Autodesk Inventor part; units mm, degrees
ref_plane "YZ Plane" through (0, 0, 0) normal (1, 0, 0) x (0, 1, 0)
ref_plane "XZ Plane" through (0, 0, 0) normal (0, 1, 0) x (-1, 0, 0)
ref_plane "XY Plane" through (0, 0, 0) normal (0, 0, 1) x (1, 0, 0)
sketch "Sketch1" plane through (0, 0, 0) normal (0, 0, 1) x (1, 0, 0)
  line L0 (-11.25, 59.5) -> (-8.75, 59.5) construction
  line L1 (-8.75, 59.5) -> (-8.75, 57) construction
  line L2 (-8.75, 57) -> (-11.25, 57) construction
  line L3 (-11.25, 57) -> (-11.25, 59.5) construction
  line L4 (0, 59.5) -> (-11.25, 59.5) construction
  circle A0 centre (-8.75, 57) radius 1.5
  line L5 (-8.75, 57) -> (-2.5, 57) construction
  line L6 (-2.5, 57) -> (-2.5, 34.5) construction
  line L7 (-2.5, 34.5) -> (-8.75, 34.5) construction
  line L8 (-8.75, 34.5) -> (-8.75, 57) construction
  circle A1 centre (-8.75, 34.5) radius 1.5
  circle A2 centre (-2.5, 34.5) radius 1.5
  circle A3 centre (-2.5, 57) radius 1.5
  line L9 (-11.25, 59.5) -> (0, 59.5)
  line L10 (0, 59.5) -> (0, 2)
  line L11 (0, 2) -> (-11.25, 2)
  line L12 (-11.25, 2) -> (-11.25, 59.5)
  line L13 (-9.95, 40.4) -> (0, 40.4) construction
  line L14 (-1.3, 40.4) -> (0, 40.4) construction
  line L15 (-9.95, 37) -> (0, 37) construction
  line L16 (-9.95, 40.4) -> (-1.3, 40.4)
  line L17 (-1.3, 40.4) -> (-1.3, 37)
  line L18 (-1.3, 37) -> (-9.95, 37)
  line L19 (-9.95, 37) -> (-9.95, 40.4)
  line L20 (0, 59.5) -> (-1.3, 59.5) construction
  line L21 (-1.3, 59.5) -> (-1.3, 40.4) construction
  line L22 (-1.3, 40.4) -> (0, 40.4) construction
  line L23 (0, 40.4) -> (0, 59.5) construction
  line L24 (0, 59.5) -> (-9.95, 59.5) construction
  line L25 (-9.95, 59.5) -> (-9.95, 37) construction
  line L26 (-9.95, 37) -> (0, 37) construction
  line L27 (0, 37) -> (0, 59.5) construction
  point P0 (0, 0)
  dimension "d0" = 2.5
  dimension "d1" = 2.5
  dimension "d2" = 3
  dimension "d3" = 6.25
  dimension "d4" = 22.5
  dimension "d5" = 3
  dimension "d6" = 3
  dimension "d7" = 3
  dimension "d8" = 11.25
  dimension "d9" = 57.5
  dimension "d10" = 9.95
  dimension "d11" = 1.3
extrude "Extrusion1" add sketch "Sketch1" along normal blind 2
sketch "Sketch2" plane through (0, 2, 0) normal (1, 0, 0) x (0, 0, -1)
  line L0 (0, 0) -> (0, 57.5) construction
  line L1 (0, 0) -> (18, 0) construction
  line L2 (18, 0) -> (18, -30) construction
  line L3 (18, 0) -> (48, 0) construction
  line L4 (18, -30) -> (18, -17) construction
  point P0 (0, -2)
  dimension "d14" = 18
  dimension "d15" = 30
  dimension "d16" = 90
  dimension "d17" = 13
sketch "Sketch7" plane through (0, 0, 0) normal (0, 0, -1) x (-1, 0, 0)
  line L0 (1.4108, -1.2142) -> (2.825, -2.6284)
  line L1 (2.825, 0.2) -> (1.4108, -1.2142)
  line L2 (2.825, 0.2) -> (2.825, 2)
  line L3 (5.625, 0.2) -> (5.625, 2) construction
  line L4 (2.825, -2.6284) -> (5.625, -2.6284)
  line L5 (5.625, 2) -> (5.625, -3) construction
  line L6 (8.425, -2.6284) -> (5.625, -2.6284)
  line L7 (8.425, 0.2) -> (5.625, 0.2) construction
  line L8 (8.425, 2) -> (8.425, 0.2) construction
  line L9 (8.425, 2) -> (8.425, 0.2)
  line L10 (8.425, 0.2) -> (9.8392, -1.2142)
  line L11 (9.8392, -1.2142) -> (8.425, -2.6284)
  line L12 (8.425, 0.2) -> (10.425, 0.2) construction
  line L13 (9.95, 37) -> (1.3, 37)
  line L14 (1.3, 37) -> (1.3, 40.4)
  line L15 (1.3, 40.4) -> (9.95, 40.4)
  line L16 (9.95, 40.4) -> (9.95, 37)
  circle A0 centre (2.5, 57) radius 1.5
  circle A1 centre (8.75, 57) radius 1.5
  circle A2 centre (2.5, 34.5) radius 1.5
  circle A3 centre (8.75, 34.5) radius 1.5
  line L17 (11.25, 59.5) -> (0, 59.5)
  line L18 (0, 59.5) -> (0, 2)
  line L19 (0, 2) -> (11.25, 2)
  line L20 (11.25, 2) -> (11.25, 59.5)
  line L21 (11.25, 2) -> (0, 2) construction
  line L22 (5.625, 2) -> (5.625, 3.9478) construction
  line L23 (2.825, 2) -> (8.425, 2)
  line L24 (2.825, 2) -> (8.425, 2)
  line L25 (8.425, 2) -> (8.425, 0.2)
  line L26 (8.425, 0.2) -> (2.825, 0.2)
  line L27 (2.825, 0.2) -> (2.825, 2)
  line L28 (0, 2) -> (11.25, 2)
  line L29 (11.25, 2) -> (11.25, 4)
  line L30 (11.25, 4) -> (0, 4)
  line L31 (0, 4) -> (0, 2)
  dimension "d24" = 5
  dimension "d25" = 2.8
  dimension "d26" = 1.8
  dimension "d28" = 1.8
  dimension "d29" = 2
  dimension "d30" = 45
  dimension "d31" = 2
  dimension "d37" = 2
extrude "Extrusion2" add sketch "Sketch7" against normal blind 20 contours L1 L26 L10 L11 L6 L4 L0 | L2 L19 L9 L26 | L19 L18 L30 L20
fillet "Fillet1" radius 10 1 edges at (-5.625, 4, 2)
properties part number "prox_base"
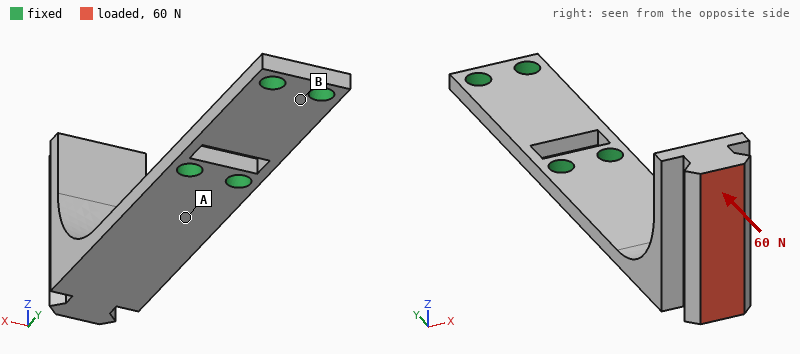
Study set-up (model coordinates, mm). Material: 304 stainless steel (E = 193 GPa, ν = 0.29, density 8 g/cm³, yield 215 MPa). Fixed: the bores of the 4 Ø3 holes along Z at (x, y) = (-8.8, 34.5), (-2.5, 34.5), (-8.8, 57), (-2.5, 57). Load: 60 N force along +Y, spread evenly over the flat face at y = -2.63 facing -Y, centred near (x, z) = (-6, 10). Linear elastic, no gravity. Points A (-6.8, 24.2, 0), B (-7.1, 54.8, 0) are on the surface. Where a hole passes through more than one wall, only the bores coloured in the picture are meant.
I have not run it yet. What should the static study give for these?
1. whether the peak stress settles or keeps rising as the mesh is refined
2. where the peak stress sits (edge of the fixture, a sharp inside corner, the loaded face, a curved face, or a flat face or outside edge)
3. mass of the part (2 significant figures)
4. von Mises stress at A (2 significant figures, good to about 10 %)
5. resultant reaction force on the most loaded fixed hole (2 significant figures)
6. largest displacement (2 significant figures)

keeps rising
edge of the fixture
19 g
67 MPa
30 N
0.26 mm
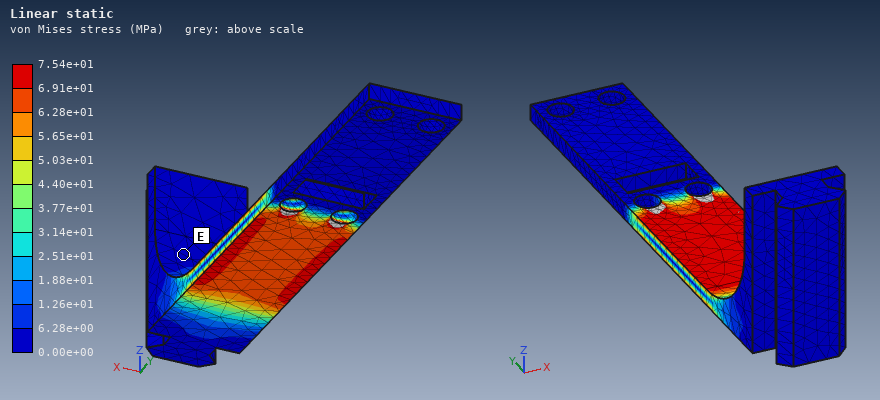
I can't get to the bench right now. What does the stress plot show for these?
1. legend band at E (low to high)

0.00e+00 to 6.28e+00 MPa
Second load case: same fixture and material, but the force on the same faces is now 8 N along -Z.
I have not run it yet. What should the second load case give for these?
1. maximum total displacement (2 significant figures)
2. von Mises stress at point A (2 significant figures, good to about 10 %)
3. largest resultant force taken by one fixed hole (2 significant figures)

0.10 mm
28 MPa
4.0 N
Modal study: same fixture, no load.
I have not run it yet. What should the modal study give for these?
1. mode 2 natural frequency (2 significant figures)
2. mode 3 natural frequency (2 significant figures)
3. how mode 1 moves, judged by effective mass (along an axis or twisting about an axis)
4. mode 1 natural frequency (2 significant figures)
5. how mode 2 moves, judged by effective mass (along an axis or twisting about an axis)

1500 Hz
3500 Hz
along Z
520 Hz
along X
